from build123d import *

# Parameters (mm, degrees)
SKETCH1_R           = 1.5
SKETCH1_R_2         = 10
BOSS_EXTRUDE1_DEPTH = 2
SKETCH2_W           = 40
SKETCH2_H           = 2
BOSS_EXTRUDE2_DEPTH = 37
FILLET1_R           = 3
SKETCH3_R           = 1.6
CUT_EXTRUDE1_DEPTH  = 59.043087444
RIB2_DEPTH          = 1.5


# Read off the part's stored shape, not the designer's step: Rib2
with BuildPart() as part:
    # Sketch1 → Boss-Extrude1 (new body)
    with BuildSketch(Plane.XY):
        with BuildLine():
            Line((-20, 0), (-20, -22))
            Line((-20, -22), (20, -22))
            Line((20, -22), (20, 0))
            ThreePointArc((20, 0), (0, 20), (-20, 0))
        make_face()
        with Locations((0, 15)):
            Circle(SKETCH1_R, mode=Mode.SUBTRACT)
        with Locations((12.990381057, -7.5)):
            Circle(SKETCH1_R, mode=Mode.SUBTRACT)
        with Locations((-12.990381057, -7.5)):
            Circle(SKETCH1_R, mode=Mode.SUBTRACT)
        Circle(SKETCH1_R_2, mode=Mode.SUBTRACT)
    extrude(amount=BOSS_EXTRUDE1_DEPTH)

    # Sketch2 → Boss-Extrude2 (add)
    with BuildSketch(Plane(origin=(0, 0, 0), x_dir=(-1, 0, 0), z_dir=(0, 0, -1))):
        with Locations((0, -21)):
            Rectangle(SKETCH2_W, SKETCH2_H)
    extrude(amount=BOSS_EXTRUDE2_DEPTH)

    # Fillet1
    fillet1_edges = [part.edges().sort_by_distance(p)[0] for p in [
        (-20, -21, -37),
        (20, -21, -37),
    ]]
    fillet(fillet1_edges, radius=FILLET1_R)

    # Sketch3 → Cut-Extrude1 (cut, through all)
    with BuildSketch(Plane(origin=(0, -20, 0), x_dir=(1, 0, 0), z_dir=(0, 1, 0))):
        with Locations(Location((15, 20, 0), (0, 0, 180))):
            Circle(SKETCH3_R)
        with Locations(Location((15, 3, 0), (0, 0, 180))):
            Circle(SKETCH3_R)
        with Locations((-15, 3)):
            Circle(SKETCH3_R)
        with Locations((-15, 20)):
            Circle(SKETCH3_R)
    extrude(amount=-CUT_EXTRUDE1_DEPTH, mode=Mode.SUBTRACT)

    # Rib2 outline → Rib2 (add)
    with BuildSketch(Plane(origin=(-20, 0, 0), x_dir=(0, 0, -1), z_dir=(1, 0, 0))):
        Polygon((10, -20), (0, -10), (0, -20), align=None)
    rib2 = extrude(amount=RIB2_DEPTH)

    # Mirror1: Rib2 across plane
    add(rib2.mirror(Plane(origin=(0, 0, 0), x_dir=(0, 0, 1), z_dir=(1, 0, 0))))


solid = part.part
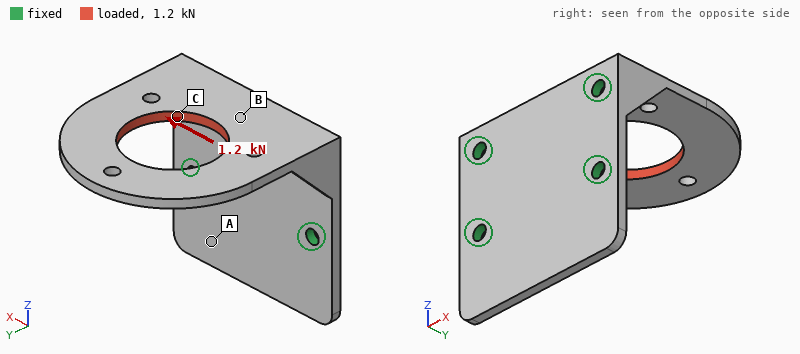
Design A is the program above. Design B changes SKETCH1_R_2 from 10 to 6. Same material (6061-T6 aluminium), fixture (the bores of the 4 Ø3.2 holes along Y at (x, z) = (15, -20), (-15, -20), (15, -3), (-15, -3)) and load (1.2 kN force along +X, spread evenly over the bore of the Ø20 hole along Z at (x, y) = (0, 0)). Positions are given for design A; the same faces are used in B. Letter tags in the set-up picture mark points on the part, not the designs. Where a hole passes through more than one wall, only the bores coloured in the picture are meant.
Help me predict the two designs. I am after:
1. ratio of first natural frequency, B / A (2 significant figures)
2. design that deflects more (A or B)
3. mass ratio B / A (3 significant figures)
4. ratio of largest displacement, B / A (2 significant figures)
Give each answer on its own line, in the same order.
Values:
1.0
A
1.07
0.79
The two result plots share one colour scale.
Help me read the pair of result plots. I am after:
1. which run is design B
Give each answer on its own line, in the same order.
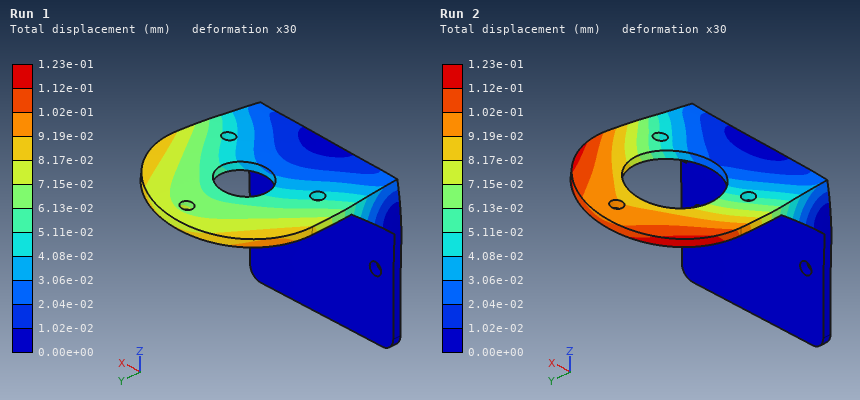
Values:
Run 1
